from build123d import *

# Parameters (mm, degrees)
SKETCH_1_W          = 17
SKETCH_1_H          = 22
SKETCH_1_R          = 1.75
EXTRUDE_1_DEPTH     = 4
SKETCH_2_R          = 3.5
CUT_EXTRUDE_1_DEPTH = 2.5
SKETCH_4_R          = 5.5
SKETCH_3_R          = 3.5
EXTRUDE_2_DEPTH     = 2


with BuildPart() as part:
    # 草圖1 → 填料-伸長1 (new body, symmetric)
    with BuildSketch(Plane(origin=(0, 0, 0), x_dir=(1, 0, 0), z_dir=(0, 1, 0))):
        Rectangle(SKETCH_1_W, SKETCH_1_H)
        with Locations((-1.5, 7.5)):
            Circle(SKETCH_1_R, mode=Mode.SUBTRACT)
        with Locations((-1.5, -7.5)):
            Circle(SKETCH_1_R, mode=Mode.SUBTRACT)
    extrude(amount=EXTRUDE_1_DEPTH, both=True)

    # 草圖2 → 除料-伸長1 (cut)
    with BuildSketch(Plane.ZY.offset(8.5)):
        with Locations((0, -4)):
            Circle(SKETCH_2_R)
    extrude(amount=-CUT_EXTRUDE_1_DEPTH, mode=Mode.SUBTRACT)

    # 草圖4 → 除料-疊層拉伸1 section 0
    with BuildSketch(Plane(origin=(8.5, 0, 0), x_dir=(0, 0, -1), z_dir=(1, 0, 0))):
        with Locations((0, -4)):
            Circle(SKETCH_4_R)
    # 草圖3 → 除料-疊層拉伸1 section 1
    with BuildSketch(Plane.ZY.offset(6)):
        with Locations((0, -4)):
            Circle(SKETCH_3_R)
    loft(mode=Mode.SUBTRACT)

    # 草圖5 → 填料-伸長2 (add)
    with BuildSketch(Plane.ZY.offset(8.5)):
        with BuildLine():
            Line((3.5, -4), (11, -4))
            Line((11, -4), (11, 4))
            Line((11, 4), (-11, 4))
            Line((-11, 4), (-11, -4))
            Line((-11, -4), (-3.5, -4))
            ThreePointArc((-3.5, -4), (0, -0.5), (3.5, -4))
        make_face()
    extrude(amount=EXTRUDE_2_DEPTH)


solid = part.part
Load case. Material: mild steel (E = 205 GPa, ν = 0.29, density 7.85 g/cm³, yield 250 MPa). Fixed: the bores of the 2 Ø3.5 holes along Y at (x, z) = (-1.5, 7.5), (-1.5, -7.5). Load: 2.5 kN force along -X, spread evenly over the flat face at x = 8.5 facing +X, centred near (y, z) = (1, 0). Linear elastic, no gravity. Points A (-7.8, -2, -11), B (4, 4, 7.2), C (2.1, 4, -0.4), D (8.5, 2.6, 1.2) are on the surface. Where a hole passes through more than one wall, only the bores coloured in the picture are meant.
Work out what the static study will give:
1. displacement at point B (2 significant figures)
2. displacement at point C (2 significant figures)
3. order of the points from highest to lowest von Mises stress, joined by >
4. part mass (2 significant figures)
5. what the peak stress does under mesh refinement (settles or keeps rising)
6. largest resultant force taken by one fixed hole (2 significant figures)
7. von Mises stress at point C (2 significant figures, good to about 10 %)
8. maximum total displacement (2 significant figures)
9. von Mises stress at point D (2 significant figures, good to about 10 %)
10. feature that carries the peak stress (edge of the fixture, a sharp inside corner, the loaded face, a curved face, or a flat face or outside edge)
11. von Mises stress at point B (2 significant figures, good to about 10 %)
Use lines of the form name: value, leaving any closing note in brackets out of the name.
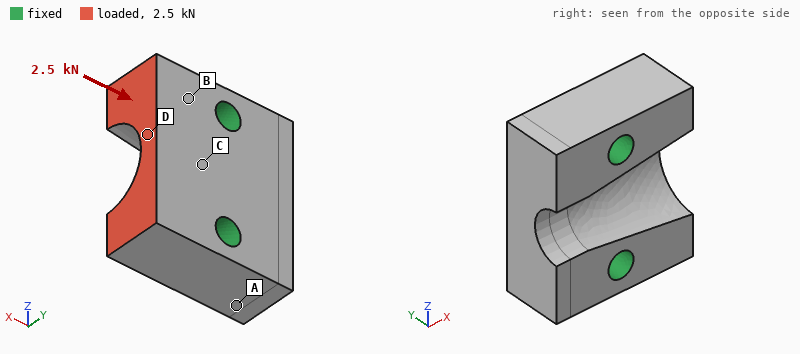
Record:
displacement at point B: 0.59 µm
displacement at point C: 0.60 µm
order of the points from highest to lowest von Mises stress, joined by >: B > D > C > A
part mass: 21 g
what the peak stress does under mesh refinement: keeps rising
largest resultant force taken by one fixed hole: 1.3 kN
von Mises stress at point C: 11 MPa
maximum total displacement: 1.2 µm
von Mises stress at point D: 17 MPa
feature that carries the peak stress: edge of the fixture
von Mises stress at point B: 24 MPa
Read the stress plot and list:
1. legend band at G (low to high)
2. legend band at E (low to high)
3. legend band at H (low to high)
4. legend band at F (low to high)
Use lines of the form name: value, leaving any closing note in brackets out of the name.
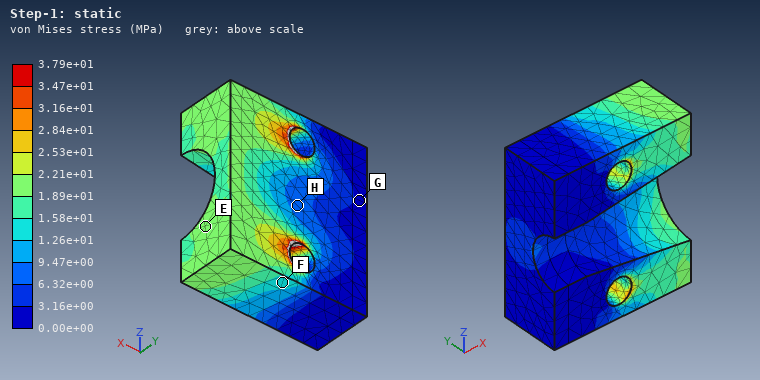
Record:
legend band at G: 0.00e+00 to 3.16e+00 MPa
legend band at E: 1.89e+01 to 2.21e+01 MPa
legend band at H: 6.32e+00 to 9.47e+00 MPa
legend band at F: 1.26e+01 to 1.58e+01 MPa
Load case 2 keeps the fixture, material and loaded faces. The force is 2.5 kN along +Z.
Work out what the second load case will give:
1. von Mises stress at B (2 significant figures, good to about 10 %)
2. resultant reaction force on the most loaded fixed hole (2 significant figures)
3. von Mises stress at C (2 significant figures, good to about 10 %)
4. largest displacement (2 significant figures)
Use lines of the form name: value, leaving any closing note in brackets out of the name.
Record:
von Mises stress at B: 33 MPa
resultant reaction force on the most loaded fixed hole: 1.7 kN
von Mises stress at C: 49 MPa
largest displacement: 6.0 µm
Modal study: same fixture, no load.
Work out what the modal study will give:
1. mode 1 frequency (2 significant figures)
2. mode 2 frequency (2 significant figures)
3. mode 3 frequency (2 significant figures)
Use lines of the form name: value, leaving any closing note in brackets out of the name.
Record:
mode 1 frequency: 51 kHz
mode 2 frequency: 58 kHz
mode 3 frequency: 59 kHz
